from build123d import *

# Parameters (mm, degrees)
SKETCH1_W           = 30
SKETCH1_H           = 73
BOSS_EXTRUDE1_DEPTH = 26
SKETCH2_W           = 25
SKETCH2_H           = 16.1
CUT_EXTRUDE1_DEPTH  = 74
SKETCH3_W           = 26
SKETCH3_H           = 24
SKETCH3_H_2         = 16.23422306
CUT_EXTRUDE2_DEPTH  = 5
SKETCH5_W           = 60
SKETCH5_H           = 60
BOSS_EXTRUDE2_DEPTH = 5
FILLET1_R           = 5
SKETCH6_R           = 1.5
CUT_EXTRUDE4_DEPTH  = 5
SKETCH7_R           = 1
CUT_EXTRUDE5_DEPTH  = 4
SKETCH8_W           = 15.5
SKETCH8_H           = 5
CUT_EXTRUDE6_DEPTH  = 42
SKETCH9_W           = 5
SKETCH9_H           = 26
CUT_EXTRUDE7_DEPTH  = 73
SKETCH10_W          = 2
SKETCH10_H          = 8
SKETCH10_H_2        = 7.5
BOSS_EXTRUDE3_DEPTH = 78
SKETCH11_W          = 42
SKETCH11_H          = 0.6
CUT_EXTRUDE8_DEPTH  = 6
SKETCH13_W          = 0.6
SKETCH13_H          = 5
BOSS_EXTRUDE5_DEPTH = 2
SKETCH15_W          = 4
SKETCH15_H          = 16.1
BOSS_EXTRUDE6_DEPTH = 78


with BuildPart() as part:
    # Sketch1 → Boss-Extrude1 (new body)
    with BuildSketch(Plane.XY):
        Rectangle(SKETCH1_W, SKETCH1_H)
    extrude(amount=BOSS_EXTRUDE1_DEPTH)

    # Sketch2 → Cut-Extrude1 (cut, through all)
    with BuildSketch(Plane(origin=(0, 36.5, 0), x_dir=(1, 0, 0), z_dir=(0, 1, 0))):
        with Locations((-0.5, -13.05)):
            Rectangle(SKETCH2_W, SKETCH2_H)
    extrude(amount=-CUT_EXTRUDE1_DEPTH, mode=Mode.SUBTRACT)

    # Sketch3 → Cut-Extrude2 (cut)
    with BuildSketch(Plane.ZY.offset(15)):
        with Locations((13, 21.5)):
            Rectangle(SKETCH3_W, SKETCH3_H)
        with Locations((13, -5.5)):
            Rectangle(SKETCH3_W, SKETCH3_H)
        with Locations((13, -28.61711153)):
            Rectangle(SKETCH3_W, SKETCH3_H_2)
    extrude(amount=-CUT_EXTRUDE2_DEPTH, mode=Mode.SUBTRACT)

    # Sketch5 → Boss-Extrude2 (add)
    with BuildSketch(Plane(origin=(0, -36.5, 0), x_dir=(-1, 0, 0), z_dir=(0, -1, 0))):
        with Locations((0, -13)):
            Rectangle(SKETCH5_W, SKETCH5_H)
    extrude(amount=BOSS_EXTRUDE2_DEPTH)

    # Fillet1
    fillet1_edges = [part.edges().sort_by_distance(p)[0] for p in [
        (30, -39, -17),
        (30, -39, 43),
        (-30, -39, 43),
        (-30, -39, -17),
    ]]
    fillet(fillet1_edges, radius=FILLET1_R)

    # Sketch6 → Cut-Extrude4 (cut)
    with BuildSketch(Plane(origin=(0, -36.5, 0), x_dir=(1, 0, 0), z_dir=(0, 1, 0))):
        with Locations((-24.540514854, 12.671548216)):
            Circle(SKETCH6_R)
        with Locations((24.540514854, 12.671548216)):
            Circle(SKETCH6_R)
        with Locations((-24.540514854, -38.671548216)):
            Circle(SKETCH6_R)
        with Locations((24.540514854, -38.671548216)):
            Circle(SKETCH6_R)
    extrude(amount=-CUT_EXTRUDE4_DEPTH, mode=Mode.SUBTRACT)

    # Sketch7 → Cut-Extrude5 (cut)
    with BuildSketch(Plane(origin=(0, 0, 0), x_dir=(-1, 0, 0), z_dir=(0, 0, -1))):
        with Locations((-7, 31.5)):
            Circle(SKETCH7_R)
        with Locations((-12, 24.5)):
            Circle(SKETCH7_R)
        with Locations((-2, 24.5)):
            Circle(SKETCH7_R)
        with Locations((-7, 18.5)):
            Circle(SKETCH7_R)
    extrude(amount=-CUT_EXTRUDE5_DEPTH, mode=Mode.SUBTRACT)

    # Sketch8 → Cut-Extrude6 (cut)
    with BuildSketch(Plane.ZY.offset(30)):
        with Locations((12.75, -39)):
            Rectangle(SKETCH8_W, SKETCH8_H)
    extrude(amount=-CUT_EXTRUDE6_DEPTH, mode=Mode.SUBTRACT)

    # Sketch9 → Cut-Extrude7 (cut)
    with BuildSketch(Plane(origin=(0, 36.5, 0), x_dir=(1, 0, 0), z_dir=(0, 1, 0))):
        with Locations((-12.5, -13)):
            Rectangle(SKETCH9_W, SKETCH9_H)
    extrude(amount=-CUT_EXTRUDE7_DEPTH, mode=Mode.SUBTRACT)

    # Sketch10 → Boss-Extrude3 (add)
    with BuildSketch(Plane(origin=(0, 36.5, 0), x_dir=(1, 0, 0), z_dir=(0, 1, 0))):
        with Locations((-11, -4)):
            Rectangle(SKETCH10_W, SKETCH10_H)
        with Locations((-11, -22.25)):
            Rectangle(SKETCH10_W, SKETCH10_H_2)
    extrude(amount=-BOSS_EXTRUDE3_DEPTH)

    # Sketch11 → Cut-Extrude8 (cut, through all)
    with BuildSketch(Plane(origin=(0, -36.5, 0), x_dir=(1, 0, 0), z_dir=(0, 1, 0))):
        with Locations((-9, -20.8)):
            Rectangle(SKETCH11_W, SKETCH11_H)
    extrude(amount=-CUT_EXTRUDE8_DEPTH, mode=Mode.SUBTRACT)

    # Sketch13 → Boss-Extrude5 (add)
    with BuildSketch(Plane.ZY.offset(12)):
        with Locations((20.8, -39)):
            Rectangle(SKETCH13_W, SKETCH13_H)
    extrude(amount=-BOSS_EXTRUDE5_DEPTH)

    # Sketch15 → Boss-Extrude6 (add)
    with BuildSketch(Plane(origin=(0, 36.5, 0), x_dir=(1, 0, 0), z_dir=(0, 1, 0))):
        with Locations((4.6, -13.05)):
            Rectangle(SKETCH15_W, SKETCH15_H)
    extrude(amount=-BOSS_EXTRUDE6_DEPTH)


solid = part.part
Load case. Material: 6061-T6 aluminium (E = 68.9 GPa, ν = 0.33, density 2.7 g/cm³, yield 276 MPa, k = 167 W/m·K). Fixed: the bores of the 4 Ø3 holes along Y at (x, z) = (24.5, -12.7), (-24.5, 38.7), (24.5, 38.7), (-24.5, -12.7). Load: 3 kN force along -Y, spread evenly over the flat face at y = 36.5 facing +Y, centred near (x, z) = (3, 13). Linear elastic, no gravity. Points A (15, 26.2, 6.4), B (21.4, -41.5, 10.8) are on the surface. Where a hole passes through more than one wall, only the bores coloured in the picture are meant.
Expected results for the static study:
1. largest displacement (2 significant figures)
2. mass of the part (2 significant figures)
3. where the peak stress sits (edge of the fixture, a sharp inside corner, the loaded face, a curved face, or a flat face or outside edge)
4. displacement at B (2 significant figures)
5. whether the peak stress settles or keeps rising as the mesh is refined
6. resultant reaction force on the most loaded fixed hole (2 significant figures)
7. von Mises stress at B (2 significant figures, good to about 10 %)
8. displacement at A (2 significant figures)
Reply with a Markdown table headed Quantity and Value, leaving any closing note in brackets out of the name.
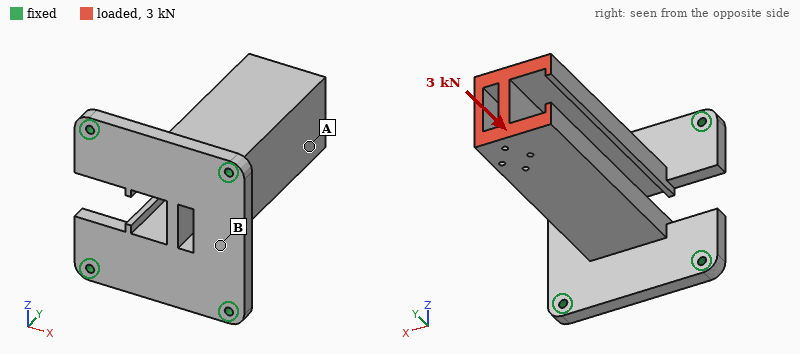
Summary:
| Quantity | Value |
|---|---|
| largest displacement | 89 µm |
| mass of the part | 120 g |
| where the peak stress sits | edge of the fixture |
| displacement at B | 48 µm |
| whether the peak stress settles or keeps rising as the mesh is refined | keeps rising |
| resultant reaction force on the most loaded fixed hole | 900 N |
| von Mises stress at B | 28 MPa |
| displacement at A | 73 µm |
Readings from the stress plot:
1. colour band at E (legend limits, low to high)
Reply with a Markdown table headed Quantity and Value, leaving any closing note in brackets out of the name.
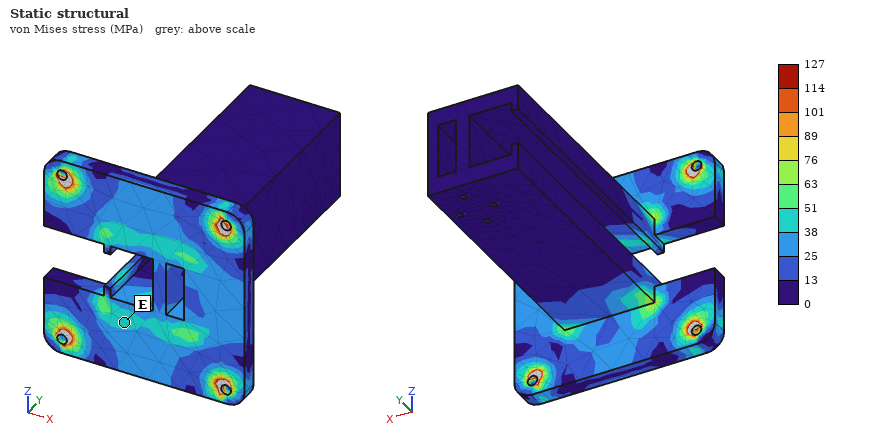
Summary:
| Quantity | Value |
|---|---|
| colour band at E | 38 to 51 MPa |
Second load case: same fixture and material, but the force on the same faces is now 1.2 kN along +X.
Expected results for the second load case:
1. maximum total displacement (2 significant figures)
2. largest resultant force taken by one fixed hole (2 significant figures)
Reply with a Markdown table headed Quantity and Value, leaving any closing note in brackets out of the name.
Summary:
| Quantity | Value |
|---|---|
| maximum total displacement | 0.52 mm |
| largest resultant force taken by one fixed hole | 1.1 kN |
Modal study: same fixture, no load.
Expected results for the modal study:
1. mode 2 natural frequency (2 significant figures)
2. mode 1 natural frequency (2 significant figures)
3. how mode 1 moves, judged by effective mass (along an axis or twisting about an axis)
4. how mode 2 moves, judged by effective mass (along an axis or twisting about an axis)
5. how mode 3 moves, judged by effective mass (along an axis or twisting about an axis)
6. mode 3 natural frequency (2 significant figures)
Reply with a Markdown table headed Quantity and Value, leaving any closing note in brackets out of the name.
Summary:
| Quantity | Value |
|---|---|
| mode 2 natural frequency | 1600 Hz |
| mode 1 natural frequency | 1500 Hz |
| how mode 1 moves, judged by effective mass | along X |
| how mode 2 moves, judged by effective mass | along Z |
| how mode 3 moves, judged by effective mass | along Y |
| mode 3 natural frequency | 3600 Hz |
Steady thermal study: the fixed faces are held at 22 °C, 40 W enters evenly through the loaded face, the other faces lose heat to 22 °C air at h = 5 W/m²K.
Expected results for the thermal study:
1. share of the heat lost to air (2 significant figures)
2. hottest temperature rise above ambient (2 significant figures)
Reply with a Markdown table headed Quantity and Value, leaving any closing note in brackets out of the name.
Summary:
| Quantity | Value |
|---|---|
| share of the heat lost to air | 6.9 % |
| hottest temperature rise above ambient | 57 K |
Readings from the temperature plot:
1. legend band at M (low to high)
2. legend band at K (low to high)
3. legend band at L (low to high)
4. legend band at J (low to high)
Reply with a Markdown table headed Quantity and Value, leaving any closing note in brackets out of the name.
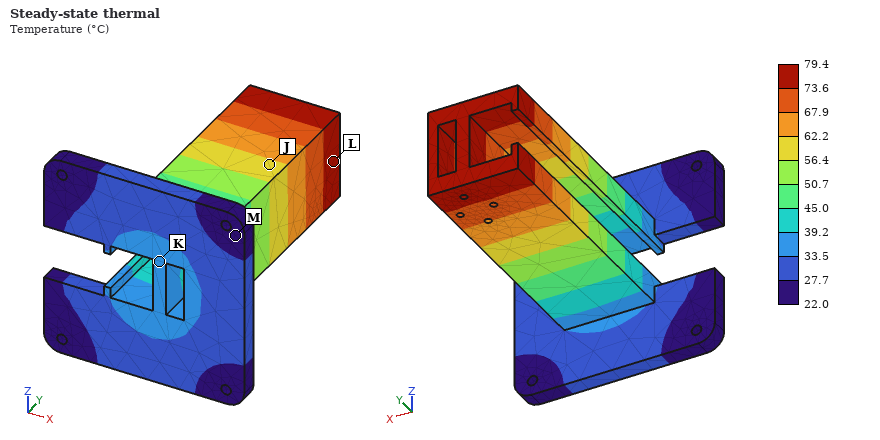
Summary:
| Quantity | Value |
|---|---|
| legend band at M | 22.0 to 27.7 °C |
| legend band at K | 33.5 to 39.2 °C |
| legend band at L | 73.6 to 79.4 °C |
| legend band at J | 56.4 to 62.2 °C |
